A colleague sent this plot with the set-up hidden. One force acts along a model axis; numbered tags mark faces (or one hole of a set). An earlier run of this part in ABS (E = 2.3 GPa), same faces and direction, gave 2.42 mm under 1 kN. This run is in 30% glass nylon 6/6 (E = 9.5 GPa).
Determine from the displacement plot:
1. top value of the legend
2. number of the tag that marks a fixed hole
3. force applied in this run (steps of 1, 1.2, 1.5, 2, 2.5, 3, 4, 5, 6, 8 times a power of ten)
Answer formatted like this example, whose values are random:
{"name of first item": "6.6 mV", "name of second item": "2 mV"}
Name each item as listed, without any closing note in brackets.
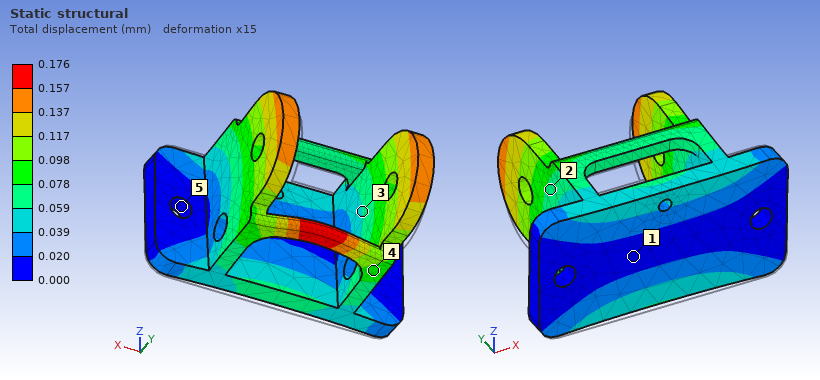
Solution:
{"top value of the legend": "0.176 mm", "number of the tag that marks a fixed hole": "5", "force applied in this run": "300 N"}
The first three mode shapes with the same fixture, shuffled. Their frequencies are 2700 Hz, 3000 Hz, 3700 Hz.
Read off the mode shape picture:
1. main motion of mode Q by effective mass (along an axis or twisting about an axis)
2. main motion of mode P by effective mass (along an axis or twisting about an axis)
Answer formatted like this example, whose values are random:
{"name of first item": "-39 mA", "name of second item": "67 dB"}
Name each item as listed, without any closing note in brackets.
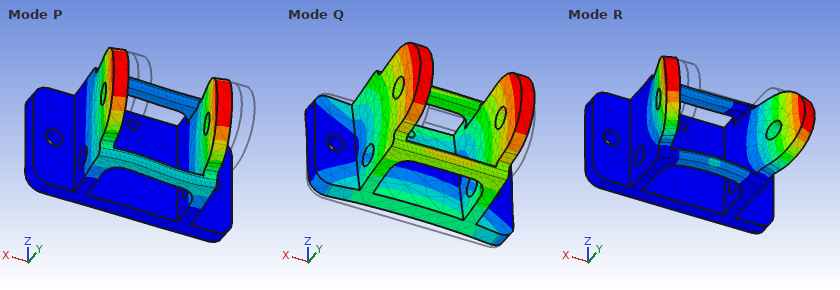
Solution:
{"main motion of mode Q by effective mass": "along Z", "main motion of mode P by effective mass": "along X"}
